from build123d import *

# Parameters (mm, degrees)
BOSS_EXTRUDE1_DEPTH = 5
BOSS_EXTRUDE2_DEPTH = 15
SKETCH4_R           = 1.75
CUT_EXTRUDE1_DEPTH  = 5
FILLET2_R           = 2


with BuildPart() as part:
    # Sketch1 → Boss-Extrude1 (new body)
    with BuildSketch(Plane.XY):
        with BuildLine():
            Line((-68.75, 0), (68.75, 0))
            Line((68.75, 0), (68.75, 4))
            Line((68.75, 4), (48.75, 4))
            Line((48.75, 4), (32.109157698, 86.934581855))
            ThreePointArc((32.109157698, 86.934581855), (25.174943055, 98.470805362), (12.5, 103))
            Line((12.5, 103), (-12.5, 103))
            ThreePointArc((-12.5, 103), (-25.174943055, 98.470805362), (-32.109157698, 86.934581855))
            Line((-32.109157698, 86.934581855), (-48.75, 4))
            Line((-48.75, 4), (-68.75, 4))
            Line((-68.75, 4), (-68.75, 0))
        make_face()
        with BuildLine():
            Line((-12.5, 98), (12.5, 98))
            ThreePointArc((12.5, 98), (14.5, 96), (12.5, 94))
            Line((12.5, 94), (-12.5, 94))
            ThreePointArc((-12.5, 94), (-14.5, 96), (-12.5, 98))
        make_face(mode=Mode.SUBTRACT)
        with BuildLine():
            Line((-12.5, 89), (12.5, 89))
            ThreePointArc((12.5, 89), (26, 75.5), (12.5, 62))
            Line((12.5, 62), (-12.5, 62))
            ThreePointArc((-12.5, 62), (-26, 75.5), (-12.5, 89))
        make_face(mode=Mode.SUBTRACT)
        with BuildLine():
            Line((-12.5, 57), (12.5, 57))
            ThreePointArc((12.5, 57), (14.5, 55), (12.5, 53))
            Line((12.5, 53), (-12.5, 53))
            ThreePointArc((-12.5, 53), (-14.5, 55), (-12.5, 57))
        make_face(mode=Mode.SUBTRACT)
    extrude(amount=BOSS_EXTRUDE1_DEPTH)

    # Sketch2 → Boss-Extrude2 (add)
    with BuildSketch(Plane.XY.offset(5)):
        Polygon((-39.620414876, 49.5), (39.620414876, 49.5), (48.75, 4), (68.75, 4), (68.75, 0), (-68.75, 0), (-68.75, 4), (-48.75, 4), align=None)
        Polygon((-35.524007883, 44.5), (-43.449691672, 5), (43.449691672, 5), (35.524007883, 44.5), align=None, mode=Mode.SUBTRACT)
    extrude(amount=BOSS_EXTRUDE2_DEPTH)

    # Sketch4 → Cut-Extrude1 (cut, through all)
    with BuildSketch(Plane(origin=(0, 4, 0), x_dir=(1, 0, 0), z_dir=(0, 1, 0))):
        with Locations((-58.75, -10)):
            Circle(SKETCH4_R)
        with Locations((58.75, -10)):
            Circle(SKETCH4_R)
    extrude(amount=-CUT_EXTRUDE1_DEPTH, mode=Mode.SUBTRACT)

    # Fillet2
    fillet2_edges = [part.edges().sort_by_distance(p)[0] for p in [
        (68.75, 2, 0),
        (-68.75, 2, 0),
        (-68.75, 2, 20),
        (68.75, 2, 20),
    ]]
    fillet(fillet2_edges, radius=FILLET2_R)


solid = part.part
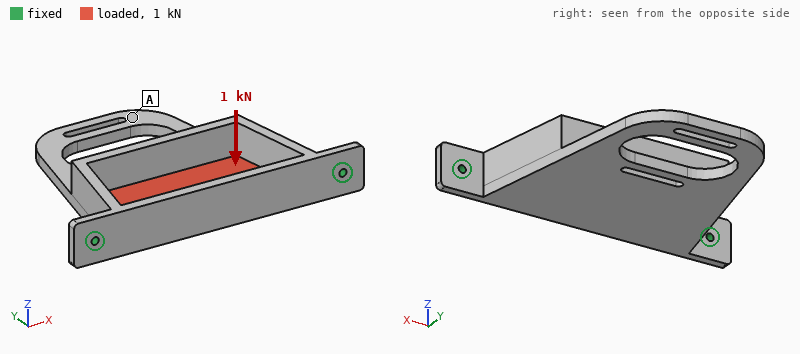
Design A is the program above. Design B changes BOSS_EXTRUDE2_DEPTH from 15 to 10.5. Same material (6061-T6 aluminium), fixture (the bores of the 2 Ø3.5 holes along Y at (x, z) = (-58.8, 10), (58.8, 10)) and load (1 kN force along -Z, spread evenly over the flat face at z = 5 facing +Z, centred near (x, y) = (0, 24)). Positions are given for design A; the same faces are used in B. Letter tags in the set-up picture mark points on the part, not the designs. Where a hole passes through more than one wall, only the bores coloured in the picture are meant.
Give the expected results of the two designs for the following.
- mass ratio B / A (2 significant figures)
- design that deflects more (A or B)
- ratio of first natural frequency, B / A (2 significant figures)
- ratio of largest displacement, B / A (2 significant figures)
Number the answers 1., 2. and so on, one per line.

1. 0.88
2. B
3. 0.87
4. 1.4
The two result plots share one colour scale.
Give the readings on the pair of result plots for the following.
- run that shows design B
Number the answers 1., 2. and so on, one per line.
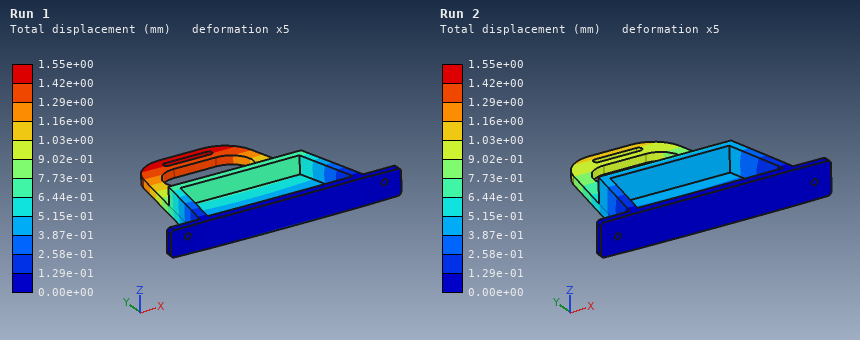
1. Run 1
